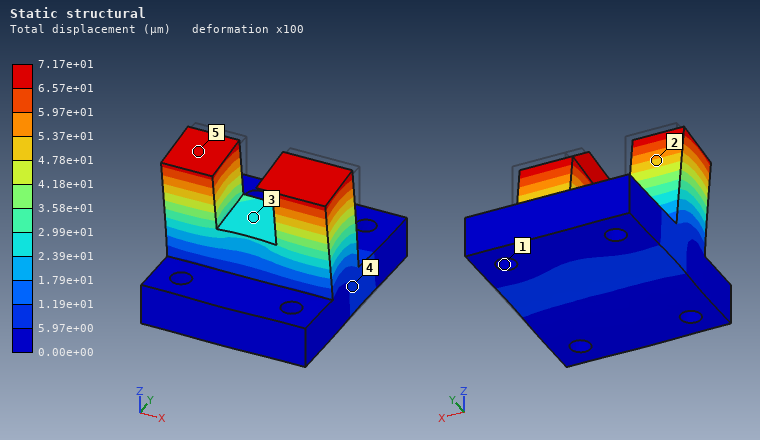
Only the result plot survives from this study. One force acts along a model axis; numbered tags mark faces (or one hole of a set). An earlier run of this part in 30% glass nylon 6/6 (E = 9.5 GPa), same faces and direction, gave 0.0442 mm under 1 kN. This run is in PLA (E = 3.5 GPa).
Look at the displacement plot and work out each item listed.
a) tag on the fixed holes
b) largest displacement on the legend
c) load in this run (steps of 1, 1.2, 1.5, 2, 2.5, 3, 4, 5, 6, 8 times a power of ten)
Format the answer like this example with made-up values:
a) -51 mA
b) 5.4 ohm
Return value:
a) 1
b) 7.17e+01 µm
c) 600 N
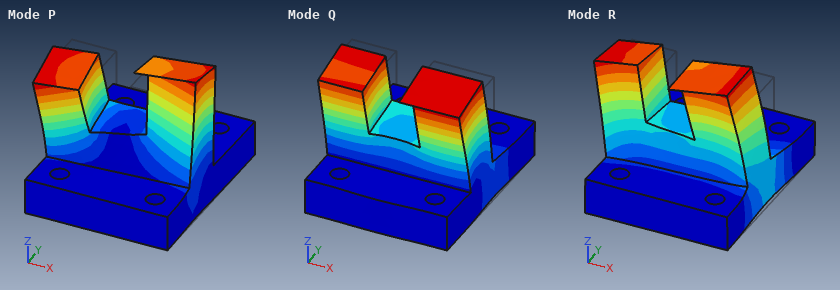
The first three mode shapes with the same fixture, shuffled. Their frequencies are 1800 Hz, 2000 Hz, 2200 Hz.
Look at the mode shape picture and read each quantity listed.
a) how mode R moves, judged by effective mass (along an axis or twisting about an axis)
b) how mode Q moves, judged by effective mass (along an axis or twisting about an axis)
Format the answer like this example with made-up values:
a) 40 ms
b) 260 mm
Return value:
a) along X
b) along Y
